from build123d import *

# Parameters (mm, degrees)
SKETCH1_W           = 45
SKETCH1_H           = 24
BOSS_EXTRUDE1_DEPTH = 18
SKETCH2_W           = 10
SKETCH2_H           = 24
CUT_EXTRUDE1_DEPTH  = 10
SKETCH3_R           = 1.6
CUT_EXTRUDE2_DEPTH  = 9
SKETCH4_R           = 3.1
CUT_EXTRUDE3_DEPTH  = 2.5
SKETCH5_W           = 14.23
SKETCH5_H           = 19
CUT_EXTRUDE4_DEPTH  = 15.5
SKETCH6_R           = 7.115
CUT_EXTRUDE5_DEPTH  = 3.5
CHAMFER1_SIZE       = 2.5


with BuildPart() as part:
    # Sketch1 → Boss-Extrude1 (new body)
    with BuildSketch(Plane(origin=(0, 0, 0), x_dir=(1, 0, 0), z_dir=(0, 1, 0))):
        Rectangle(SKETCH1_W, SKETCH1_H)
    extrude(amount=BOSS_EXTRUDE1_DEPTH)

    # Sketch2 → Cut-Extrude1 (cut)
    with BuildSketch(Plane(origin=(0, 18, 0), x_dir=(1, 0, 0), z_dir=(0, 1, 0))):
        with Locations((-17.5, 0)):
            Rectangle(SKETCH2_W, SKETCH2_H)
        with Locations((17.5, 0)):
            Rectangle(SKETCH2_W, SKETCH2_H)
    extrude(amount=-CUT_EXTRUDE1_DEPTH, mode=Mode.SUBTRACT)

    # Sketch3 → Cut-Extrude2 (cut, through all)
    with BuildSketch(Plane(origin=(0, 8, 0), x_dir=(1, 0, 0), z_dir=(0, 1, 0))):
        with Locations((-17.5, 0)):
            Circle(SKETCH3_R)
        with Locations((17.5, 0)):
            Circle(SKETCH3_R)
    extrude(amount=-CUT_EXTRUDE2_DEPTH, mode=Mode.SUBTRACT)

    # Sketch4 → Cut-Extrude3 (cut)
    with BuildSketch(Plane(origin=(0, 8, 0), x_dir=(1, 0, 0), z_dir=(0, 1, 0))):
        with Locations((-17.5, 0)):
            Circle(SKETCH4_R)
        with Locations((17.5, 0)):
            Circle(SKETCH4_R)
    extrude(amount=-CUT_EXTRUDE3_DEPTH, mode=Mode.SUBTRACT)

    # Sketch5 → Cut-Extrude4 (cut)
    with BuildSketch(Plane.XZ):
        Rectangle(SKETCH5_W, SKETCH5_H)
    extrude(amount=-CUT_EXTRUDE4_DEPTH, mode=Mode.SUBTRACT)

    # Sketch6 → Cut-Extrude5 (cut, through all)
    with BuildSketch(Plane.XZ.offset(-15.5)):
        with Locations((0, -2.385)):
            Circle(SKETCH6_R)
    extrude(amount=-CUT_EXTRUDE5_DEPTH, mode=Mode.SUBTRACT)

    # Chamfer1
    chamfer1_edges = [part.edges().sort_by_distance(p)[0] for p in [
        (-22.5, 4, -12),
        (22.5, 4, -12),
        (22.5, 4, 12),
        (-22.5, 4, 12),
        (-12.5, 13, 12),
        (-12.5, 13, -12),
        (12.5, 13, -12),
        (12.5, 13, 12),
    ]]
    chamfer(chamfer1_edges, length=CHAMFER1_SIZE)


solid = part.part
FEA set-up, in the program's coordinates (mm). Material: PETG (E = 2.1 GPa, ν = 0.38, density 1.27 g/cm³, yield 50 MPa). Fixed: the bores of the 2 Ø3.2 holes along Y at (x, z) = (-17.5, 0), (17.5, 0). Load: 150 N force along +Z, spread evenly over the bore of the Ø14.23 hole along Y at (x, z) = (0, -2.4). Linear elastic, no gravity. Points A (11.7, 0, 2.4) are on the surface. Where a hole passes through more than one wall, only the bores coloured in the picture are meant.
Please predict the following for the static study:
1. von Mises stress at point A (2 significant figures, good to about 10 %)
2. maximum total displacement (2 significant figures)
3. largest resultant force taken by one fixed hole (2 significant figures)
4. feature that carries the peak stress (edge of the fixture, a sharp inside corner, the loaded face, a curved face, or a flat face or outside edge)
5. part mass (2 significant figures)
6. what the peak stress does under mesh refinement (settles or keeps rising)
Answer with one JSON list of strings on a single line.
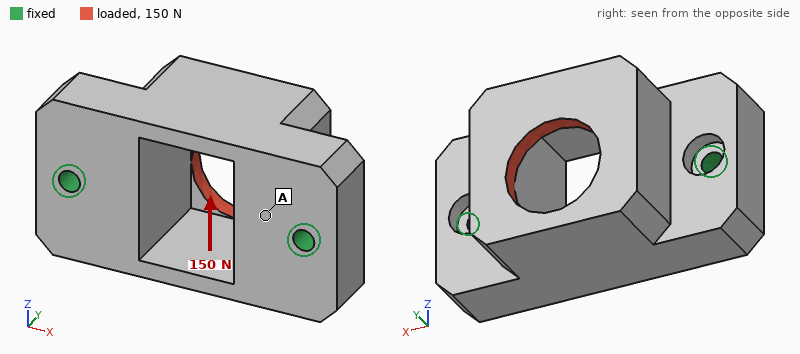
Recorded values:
["1.9 MPa", "0.20 mm", "75 N", "edge of the fixture", "12 g", "keeps rising"]
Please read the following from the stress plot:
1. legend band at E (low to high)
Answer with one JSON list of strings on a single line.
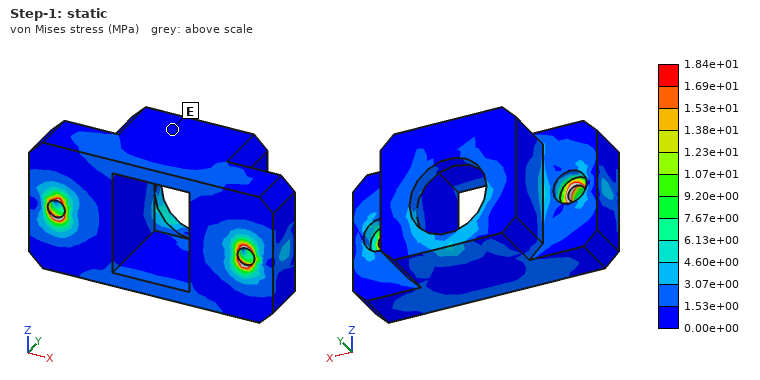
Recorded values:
["0.00e+00 to 1.53e+00 MPa"]
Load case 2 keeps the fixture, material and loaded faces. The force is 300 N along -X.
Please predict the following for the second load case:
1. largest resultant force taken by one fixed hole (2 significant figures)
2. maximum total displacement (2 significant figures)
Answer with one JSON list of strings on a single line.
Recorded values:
["190 N", "78 µm"]
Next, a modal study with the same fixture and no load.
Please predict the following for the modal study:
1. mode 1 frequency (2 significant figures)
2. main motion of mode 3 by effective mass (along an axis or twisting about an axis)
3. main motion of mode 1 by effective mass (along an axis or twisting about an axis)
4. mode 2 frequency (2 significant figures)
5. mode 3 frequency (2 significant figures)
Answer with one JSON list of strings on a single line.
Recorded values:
["2400 Hz", "along Y", "along Z", "4400 Hz", "5000 Hz"]
